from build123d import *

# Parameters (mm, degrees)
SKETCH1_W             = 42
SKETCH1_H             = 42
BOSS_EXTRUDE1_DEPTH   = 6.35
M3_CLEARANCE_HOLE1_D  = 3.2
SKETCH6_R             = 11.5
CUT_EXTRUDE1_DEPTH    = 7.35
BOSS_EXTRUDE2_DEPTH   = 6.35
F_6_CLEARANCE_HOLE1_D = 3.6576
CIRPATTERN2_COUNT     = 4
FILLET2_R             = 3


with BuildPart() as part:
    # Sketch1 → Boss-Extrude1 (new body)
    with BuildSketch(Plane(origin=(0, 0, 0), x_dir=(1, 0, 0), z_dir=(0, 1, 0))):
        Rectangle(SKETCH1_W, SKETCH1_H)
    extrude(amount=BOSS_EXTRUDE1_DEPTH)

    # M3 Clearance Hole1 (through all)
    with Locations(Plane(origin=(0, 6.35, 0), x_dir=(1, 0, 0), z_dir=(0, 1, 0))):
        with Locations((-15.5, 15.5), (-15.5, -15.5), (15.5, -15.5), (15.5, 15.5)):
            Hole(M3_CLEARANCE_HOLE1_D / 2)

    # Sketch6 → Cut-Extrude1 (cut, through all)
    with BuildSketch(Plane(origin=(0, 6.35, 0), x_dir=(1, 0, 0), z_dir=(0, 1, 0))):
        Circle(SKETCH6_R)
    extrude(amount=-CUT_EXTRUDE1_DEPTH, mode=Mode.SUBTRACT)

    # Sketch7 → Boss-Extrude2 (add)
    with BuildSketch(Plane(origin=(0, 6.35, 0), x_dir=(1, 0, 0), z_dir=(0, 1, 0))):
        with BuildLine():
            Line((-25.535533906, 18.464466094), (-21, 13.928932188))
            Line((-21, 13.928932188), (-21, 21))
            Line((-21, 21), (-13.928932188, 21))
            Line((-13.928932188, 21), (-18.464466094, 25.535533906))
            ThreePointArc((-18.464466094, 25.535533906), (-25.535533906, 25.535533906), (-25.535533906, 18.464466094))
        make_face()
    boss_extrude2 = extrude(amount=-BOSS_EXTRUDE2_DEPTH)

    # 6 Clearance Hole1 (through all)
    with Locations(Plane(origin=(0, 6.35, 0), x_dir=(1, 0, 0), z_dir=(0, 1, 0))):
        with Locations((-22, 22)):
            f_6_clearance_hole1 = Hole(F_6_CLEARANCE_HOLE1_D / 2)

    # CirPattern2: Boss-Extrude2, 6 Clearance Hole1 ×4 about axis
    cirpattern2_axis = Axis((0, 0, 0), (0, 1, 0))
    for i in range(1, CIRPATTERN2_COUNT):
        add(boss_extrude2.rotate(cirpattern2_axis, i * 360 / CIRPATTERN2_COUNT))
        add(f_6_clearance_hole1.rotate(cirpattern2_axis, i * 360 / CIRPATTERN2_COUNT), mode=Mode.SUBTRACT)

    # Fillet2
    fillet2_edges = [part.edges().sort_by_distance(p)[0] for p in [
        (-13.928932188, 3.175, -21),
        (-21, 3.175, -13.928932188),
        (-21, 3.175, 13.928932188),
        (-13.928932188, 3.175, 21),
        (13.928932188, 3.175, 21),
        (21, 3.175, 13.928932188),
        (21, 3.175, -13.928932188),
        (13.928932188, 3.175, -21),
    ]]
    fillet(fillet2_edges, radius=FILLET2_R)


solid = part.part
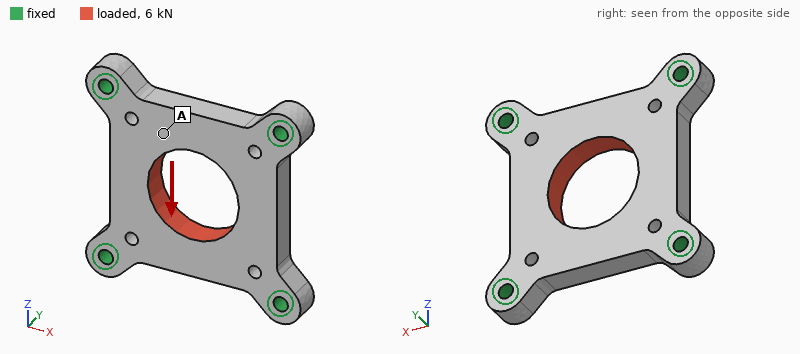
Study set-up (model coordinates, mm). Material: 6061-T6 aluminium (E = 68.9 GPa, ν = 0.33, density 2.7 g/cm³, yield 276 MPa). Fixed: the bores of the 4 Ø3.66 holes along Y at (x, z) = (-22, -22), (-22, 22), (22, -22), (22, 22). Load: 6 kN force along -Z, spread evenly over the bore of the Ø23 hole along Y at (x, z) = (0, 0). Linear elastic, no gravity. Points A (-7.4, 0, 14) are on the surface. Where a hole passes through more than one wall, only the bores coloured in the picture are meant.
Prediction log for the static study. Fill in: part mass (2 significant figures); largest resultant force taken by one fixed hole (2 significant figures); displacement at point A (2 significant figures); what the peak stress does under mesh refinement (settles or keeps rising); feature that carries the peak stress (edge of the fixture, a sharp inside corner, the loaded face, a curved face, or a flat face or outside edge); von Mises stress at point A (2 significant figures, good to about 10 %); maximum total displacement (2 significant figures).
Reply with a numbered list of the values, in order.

1. 27 g
2. 1.8 kN
3. 12 µm
4. keeps rising
5. edge of the fixture
6. 23 MPa
7. 15 µm
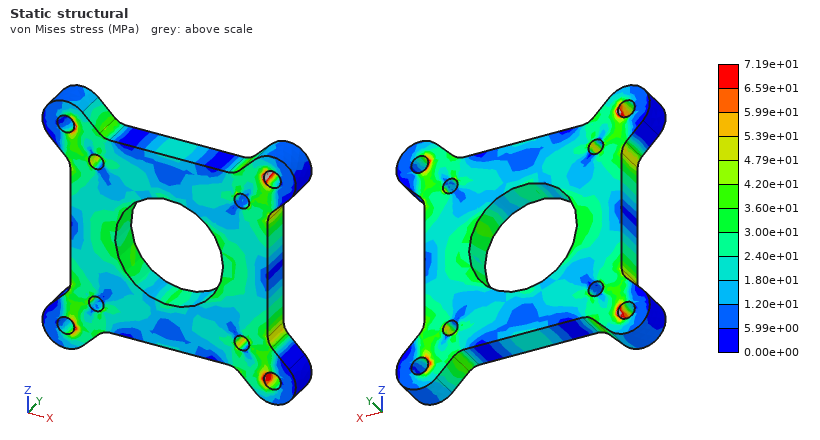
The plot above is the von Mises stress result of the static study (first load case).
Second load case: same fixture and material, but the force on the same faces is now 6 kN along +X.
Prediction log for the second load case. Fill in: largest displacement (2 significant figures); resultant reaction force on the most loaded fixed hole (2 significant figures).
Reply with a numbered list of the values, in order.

1. 15 µm
2. 1.8 kN
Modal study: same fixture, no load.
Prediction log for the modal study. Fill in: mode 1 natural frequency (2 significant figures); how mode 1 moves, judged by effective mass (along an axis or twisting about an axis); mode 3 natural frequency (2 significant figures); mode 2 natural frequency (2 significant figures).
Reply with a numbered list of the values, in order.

1. 11 kHz
2. along Y
3. 16 kHz
4. 16 kHz
